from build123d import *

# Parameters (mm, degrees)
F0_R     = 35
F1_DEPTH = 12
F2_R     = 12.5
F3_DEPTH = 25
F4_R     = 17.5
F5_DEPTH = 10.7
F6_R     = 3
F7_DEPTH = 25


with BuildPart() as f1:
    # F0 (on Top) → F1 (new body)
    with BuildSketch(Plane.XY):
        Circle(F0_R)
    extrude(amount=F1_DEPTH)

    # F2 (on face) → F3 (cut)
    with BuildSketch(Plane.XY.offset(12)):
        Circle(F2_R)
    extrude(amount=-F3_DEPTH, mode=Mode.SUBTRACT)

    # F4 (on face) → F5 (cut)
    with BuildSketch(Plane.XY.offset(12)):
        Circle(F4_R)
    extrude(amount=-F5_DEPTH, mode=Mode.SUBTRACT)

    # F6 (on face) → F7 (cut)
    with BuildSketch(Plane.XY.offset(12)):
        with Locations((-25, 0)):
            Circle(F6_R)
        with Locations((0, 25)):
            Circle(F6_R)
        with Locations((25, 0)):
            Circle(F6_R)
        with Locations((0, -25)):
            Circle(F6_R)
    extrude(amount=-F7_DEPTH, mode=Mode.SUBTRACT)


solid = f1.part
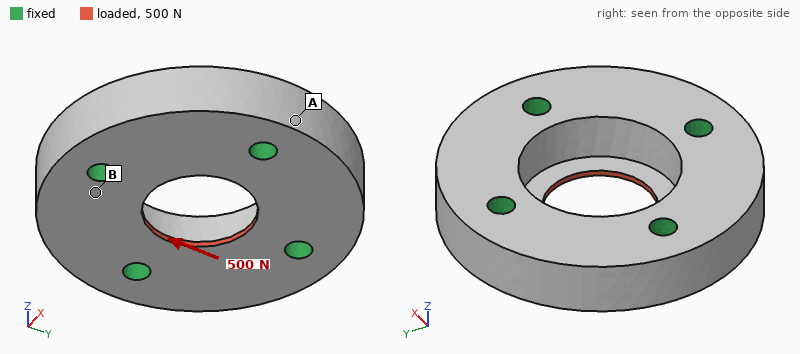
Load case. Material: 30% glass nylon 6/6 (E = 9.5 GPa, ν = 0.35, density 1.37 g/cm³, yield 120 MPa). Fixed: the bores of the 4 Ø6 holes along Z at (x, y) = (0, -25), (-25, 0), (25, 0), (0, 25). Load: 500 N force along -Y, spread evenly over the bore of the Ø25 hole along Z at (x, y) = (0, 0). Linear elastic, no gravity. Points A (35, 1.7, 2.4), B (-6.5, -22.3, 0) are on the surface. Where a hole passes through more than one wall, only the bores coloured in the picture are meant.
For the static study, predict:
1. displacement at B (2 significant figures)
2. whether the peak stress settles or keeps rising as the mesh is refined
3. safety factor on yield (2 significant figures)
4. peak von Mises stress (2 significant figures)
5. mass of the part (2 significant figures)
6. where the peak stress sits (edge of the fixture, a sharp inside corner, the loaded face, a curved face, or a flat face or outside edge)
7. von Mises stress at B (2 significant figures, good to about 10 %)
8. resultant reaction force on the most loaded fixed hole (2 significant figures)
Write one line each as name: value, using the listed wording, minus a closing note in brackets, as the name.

displacement at B: 1.3 µm
whether the peak stress settles or keeps rising as the mesh is refined: settles
safety factor on yield: 13
peak von Mises stress: 9.2 MPa
mass of the part: 46 g
where the peak stress sits: the loaded face
von Mises stress at B: 1.5 MPa
resultant reaction force on the most loaded fixed hole: 130 N
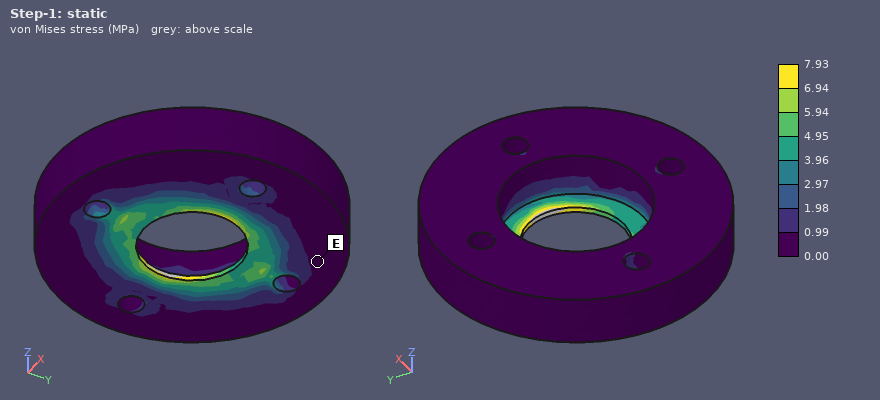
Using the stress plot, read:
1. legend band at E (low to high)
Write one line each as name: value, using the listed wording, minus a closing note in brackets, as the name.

legend band at E: 0.00 to 0.99 MPa
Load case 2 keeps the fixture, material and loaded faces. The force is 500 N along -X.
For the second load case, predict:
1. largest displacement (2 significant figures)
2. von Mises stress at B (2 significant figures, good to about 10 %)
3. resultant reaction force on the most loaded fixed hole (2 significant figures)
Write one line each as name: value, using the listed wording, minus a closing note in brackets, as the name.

largest displacement: 7.7 µm
von Mises stress at B: 0.96 MPa
resultant reaction force on the most loaded fixed hole: 130 N
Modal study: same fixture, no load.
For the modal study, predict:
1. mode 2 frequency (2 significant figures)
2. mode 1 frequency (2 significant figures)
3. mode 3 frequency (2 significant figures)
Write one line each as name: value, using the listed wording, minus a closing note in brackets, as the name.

mode 2 frequency: 12 kHz
mode 1 frequency: 11 kHz
mode 3 frequency: 12 kHz
